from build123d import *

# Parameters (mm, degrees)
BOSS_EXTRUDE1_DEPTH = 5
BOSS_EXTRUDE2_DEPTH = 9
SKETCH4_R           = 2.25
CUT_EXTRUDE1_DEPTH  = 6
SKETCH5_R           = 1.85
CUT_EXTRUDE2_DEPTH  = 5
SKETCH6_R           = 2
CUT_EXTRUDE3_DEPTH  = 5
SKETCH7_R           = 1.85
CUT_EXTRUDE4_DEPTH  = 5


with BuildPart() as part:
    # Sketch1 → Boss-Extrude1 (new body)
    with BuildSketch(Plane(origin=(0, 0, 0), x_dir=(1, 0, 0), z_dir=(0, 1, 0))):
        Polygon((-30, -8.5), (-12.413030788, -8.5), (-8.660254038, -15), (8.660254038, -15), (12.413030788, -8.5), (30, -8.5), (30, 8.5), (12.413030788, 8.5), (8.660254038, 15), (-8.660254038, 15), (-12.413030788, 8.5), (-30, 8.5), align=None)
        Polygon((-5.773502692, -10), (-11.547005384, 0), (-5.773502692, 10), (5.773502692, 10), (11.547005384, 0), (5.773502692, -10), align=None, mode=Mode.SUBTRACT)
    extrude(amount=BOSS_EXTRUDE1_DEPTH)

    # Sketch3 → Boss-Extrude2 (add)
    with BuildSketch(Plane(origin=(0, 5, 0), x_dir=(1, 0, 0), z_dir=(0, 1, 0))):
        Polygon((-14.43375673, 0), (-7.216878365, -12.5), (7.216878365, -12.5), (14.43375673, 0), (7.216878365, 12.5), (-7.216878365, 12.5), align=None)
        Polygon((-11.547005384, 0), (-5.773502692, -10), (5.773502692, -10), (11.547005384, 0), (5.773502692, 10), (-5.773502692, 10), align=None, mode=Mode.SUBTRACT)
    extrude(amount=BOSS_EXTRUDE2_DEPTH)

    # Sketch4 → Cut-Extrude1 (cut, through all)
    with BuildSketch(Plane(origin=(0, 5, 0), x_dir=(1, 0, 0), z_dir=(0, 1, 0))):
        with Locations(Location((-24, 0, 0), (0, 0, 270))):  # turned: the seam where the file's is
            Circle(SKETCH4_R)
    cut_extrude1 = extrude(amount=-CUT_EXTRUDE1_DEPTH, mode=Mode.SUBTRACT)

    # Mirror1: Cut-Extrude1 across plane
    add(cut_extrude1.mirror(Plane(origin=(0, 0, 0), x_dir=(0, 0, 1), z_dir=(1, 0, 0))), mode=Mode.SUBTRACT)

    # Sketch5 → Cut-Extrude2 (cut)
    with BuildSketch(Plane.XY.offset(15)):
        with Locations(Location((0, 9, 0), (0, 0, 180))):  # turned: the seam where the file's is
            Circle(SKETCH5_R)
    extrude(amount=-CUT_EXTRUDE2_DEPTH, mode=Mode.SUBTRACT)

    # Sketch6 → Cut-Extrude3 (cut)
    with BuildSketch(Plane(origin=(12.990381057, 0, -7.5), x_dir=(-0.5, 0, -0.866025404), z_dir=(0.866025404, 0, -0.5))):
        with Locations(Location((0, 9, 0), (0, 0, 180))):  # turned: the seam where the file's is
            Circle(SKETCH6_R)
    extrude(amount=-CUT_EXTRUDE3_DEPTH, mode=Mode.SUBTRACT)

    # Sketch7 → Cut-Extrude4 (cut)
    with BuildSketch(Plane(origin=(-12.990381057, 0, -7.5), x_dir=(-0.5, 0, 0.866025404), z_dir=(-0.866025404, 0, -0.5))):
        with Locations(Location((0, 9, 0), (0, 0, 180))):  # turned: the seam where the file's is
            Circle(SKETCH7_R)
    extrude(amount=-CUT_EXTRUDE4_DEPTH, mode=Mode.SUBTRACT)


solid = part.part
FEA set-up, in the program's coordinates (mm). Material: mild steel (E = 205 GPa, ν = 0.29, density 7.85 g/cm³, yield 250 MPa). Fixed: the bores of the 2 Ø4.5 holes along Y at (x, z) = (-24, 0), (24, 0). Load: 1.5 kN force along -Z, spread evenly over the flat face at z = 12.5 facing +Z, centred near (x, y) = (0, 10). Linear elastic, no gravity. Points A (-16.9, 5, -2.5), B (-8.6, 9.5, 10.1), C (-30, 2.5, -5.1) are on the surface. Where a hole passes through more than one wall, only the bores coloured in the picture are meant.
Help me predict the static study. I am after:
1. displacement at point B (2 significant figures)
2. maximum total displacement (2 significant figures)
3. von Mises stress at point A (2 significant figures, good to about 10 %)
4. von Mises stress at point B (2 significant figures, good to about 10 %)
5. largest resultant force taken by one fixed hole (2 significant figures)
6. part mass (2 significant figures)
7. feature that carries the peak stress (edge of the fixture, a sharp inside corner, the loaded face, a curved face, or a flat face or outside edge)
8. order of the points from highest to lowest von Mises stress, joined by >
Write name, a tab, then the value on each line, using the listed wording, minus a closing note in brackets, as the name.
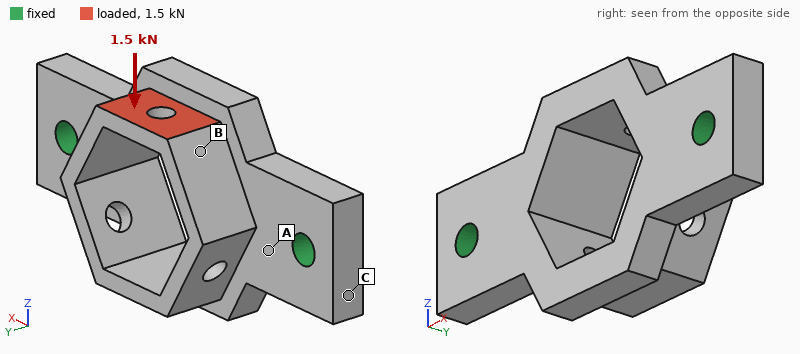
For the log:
displacement at point B	25 µm
maximum total displacement	46 µm
von Mises stress at point A	82 MPa
von Mises stress at point B	43 MPa
largest resultant force taken by one fixed hole	880 N
part mass	49 g
feature that carries the peak stress	the loaded face
order of the points from highest to lowest von Mises stress, joined by >	A > B > C
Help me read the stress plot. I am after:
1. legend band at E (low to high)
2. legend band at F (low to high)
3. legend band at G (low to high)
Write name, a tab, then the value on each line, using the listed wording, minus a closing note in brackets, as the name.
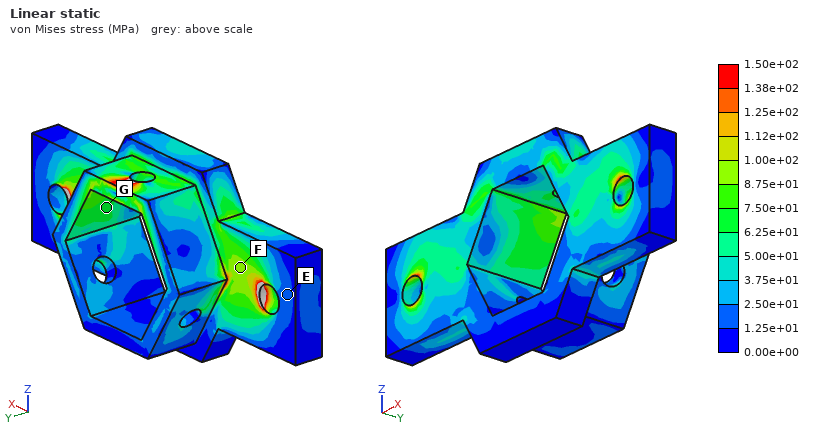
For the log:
legend band at E	1.25e+01 to 2.50e+01 MPa
legend band at F	8.75e+01 to 1.00e+02 MPa
legend band at G	6.25e+01 to 7.50e+01 MPa
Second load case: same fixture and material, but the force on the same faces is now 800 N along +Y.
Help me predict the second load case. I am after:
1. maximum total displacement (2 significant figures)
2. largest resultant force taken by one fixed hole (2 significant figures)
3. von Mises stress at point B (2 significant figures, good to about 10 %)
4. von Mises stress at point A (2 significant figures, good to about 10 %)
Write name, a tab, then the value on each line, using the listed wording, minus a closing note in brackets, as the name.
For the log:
maximum total displacement	39 µm
largest resultant force taken by one fixed hole	440 N
von Mises stress at point B	46 MPa
von Mises stress at point A	61 MPa
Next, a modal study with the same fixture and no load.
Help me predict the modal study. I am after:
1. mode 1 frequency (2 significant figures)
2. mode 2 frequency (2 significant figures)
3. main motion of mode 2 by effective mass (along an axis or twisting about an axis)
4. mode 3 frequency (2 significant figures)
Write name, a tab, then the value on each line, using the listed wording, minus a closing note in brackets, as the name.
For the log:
mode 1 frequency	7400 Hz
mode 2 frequency	9200 Hz
main motion of mode 2 by effective mass	along Y
mode 3 frequency	17 kHz
